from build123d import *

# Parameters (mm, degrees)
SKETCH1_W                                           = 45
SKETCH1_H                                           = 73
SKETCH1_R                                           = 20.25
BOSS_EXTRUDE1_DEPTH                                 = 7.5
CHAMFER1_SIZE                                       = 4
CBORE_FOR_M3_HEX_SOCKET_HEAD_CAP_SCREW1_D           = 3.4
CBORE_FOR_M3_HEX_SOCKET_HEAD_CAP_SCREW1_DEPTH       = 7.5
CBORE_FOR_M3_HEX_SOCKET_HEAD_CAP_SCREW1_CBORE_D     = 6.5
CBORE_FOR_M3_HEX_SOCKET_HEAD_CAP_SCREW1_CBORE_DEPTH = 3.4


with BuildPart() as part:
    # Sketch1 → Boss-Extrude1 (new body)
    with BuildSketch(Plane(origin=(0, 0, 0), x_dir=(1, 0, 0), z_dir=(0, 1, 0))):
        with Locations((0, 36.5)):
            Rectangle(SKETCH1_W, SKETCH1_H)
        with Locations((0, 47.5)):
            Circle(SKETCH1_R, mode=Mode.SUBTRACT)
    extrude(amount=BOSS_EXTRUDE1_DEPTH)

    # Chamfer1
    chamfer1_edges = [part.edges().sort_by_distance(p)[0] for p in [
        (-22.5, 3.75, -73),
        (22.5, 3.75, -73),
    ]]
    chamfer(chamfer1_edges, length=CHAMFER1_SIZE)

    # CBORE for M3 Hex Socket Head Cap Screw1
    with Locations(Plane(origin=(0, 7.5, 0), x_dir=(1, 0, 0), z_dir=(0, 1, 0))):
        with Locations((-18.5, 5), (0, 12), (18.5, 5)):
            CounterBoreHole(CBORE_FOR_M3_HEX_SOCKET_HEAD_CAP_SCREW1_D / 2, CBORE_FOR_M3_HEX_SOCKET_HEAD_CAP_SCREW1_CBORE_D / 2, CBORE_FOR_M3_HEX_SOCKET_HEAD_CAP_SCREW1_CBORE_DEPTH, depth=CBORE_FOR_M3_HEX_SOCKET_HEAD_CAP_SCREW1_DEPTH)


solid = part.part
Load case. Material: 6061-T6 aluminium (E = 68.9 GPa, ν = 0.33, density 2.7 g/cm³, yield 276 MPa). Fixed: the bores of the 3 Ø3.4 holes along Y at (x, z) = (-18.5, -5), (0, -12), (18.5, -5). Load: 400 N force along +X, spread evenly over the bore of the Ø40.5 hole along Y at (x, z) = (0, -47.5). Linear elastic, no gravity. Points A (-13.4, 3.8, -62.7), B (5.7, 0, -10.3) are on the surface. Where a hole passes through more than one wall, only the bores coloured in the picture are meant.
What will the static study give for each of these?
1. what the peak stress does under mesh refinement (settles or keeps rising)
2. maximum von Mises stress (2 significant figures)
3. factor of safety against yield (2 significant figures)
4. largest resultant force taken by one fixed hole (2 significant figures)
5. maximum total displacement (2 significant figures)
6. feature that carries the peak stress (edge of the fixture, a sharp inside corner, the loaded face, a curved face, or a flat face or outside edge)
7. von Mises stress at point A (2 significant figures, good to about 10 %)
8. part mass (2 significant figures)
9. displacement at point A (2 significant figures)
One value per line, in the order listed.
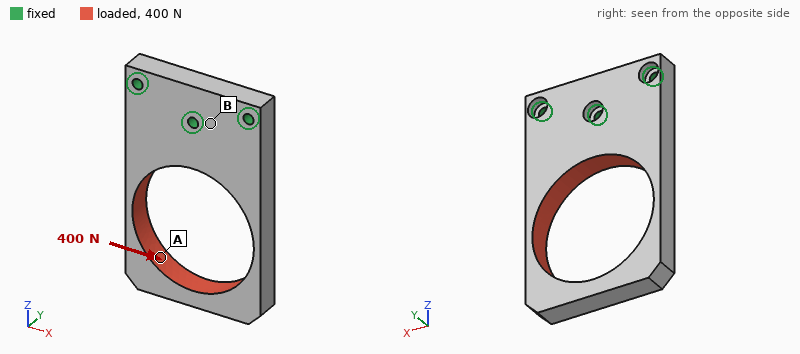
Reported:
settles
54 MPa
5.2
380 N
88 µm
the loaded face
12 MPa
39 g
83 µm
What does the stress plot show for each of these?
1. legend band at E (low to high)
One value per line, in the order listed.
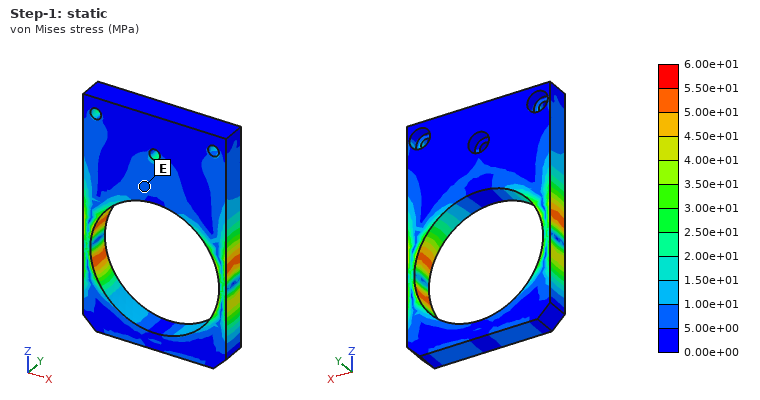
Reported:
5.00e+00 to 1.00e+01 MPa
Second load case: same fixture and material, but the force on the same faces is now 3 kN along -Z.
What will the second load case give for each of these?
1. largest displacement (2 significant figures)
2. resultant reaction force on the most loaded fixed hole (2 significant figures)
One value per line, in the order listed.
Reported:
100 µm
1.1 kN
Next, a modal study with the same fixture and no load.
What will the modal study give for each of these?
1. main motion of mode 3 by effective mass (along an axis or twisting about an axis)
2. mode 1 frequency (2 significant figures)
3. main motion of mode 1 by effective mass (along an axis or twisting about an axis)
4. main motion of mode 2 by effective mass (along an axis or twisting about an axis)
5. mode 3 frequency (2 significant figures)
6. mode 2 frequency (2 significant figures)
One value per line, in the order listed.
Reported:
twisting about Z
1200 Hz
along Y
along X
2900 Hz
2500 Hz
